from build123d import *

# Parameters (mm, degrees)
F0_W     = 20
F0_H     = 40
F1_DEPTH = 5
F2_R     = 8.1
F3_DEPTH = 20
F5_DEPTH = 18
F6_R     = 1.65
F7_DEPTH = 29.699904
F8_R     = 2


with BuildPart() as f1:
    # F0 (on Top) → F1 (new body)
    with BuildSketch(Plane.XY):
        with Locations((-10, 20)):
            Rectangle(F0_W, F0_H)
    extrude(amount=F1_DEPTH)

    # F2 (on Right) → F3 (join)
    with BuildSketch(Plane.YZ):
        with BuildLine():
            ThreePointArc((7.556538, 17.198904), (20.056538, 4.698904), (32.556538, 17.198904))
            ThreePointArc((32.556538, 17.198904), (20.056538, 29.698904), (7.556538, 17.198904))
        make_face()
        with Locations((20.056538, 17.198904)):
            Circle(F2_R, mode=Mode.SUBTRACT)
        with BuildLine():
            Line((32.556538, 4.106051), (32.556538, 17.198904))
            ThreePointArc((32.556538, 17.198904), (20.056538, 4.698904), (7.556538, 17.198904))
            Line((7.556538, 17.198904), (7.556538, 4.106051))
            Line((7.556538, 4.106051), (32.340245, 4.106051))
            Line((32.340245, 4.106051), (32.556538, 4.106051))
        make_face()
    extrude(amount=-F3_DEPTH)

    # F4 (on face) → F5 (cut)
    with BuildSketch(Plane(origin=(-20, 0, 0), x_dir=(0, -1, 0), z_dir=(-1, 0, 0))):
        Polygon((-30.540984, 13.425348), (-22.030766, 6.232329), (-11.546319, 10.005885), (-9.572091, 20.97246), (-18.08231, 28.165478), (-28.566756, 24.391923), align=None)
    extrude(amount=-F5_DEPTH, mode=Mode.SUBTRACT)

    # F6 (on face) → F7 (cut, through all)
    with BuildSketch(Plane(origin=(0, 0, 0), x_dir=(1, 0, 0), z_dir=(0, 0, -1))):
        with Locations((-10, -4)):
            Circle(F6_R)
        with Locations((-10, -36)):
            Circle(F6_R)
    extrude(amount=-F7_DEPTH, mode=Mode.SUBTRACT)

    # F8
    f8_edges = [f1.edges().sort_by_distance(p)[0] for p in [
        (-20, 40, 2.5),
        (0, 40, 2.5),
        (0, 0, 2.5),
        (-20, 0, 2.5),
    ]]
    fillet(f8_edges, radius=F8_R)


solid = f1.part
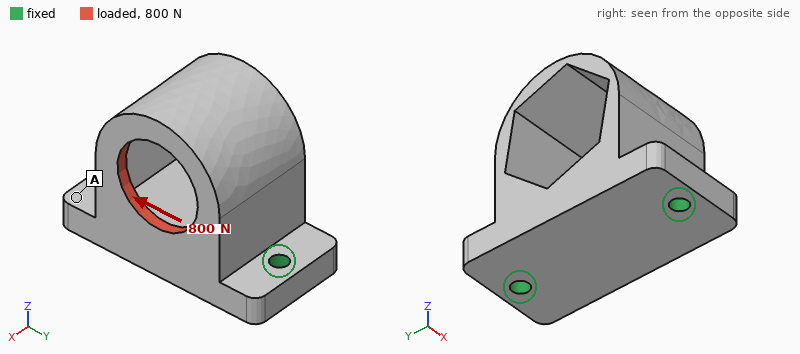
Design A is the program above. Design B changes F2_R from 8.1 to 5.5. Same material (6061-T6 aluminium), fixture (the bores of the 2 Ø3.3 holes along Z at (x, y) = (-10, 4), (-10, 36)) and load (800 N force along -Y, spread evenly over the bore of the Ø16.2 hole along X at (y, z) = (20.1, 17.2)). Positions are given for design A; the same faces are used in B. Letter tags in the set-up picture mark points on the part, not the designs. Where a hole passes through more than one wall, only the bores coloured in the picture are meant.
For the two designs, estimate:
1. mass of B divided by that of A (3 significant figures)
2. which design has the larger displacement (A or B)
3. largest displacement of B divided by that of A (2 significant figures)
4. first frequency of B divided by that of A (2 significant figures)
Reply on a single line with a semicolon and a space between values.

1.03; A; 0.59; 0.97
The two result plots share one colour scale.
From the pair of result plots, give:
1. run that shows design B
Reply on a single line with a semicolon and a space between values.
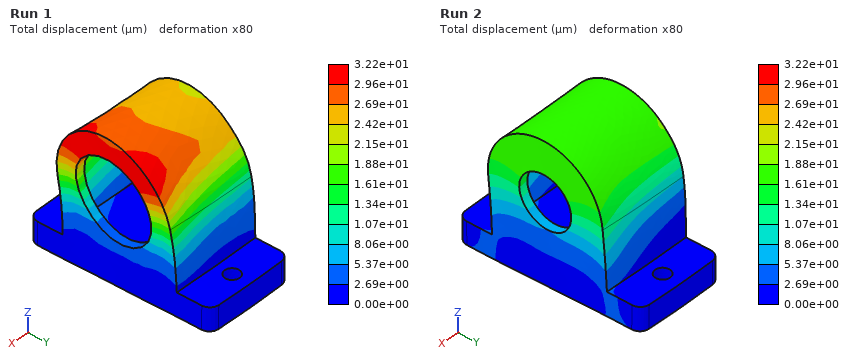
Run 2
